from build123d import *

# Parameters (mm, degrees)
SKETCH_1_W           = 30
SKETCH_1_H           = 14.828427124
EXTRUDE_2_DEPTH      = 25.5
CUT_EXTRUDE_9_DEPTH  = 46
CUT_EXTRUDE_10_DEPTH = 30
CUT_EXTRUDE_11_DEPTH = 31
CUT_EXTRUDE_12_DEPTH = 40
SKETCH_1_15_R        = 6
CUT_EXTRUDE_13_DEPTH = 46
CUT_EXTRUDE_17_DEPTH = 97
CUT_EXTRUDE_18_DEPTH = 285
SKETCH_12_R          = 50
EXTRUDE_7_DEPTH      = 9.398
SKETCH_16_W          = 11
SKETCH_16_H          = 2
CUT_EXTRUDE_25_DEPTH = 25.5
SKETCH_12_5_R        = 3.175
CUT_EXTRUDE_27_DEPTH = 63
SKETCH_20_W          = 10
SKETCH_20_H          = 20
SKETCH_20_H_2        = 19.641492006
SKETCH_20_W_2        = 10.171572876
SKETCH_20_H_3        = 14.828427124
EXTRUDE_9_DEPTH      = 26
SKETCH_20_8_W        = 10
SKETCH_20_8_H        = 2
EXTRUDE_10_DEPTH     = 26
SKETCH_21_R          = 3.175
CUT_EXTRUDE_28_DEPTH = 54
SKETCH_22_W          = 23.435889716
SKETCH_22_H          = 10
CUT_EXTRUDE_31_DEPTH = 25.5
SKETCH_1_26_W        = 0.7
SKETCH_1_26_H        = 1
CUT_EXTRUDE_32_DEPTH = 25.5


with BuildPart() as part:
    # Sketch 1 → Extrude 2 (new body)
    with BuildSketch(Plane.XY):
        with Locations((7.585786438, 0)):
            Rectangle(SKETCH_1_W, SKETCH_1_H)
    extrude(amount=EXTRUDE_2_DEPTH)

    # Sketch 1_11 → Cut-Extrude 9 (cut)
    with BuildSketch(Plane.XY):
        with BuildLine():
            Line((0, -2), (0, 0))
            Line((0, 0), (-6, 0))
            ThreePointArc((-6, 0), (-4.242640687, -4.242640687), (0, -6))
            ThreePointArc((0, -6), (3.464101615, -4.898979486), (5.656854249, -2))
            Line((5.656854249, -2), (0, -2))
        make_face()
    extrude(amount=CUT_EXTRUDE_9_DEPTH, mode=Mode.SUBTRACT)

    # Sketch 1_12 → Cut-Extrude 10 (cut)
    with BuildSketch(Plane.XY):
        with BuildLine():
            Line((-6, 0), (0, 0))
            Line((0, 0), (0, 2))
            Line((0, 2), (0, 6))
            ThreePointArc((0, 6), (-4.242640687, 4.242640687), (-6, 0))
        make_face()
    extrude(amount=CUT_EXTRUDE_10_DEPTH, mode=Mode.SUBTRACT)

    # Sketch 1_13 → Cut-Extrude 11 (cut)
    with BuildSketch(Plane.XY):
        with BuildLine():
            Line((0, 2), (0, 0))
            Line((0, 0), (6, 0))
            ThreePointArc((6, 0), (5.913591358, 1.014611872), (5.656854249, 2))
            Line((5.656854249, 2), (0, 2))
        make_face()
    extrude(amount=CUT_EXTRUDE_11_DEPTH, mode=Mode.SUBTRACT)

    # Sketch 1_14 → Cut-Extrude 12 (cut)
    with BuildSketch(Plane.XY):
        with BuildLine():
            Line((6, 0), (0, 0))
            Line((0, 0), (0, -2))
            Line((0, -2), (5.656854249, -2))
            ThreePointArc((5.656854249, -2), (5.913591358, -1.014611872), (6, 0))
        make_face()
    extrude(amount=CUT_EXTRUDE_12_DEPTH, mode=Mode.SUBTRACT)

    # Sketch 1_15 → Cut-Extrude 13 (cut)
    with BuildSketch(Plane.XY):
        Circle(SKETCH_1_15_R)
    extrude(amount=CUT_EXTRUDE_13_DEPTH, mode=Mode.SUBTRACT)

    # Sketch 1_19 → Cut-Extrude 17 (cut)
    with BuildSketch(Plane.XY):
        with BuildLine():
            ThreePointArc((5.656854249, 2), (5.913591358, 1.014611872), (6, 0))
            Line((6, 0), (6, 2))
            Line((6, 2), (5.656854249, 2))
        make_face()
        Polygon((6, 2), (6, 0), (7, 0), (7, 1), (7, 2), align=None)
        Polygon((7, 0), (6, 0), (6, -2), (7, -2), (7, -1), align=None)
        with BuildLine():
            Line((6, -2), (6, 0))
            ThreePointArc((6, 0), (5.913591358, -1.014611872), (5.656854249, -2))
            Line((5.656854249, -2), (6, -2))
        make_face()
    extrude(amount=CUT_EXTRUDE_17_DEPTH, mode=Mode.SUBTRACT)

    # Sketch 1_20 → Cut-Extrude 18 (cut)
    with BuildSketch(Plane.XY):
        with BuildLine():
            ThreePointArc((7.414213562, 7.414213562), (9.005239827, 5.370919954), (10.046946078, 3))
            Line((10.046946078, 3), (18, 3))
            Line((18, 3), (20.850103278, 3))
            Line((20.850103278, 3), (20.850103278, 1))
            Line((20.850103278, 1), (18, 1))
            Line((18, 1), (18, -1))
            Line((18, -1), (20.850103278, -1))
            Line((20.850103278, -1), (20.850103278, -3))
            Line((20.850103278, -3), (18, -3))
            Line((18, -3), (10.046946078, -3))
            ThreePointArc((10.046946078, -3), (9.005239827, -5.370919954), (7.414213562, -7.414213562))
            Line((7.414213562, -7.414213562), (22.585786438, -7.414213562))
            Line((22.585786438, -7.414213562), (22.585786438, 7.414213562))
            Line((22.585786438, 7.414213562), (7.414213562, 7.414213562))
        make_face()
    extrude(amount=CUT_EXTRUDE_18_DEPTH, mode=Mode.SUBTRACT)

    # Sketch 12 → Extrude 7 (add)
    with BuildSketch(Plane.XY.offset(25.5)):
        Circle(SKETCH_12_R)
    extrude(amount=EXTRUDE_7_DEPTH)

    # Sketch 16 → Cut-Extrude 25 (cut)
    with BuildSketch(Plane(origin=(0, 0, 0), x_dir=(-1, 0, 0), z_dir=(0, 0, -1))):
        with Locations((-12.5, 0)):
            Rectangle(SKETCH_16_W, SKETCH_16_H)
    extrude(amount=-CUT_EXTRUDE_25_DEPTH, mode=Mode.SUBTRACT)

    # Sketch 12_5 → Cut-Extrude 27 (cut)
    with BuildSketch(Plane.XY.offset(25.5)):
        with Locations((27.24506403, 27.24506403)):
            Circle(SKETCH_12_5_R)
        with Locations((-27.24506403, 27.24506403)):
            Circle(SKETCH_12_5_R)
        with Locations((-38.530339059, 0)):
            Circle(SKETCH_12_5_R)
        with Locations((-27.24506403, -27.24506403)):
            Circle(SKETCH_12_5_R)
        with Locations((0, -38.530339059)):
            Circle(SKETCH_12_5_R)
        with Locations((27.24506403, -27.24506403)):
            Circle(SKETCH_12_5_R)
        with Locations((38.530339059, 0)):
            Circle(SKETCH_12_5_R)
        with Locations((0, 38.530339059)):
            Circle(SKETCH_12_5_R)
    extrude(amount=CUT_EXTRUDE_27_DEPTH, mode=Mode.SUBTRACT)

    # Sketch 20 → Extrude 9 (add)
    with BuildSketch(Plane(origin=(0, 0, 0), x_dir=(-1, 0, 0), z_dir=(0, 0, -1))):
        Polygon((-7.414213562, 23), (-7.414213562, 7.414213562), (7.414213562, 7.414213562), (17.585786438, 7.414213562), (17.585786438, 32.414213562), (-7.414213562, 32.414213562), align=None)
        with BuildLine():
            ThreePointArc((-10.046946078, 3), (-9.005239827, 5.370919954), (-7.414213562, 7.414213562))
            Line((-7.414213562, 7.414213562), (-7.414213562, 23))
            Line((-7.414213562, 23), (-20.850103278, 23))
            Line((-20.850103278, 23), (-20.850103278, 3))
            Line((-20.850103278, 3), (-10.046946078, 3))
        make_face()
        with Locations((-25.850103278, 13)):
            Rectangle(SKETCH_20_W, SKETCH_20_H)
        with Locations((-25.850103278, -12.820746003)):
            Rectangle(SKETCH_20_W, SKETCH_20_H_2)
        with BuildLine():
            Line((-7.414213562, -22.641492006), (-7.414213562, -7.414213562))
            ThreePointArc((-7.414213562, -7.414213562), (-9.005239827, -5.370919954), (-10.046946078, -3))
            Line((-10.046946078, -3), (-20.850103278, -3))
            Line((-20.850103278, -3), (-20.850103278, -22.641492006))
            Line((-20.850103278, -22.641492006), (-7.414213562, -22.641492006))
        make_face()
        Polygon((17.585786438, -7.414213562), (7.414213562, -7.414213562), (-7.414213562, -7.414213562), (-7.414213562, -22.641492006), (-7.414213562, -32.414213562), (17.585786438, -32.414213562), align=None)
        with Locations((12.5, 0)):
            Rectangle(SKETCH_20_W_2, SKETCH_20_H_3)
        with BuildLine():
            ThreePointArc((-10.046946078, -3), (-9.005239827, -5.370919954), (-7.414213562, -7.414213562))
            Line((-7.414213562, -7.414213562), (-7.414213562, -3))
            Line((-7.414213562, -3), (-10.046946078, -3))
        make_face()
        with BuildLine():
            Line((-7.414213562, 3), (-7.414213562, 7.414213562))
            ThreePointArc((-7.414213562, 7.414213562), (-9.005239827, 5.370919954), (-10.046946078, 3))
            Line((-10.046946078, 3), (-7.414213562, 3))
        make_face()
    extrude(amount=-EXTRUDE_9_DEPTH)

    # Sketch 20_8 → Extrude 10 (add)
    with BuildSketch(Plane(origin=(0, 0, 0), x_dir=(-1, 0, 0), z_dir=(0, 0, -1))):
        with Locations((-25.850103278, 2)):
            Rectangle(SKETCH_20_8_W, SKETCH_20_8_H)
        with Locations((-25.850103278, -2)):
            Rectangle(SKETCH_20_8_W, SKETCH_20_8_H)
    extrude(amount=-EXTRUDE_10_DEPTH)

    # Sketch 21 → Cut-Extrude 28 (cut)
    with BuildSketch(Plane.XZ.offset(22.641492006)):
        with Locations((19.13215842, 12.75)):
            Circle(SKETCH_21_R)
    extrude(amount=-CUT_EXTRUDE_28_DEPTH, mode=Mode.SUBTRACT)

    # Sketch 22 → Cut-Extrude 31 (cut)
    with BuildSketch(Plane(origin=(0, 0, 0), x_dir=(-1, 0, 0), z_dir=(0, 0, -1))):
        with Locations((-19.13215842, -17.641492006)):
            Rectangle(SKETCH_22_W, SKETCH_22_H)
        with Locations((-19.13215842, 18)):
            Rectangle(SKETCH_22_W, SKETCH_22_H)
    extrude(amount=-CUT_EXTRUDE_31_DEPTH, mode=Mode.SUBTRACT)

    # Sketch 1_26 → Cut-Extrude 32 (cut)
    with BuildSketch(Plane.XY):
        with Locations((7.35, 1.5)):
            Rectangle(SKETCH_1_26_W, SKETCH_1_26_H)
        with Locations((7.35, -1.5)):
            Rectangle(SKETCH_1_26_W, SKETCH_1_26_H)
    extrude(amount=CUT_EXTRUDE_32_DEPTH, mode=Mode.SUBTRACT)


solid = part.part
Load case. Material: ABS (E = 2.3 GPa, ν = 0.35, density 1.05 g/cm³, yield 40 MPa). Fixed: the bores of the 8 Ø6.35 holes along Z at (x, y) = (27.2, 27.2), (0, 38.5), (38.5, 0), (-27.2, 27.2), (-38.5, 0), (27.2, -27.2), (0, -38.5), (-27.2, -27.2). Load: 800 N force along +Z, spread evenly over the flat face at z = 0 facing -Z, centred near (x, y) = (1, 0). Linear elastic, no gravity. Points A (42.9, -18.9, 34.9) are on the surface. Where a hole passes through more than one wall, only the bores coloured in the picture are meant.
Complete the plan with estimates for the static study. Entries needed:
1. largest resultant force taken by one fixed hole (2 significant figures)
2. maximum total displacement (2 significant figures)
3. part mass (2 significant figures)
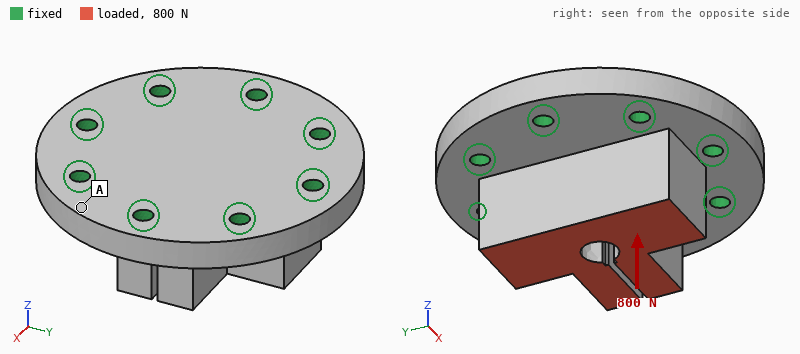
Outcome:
160 N
28 µm
130 g
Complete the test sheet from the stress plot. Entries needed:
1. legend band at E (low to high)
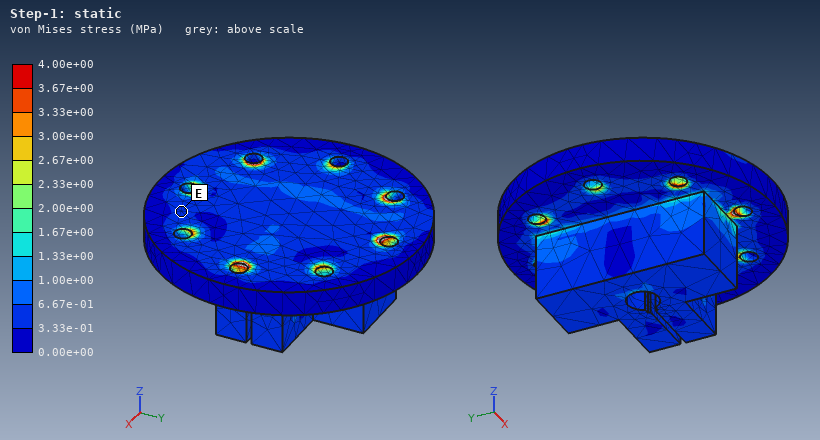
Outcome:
3.33e-01 to 6.67e-01 MPa
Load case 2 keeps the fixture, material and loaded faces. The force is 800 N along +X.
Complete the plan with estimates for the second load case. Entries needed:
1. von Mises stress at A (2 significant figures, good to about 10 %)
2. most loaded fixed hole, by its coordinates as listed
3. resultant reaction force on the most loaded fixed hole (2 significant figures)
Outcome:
0.59 MPa
(38.5, 0)
320 N
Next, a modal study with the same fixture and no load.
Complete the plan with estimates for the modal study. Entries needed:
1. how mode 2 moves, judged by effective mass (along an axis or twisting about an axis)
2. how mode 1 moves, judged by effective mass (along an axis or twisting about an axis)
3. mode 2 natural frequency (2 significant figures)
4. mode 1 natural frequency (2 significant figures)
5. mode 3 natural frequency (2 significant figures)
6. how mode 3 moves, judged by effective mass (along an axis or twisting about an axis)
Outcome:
along X
along Z
3800 Hz
3300 Hz
4000 Hz
along Y
